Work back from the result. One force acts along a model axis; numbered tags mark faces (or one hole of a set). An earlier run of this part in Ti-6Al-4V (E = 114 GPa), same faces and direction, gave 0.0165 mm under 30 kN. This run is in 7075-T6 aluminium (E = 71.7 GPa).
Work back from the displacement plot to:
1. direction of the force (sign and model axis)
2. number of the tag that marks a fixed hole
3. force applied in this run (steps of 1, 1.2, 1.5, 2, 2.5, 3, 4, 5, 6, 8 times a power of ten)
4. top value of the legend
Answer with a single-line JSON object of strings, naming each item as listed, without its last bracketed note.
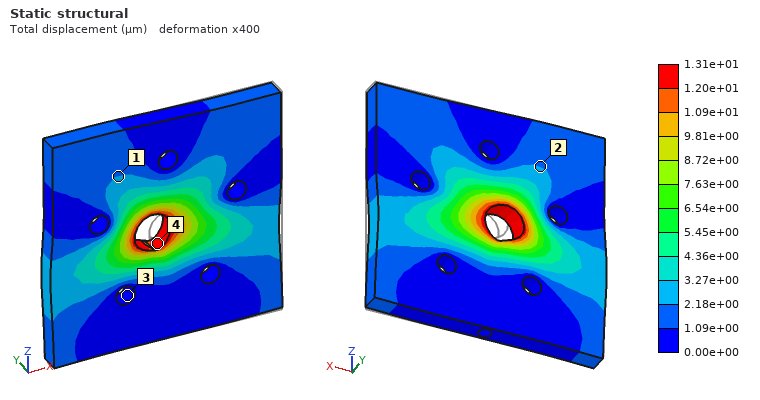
{"direction of the force": "-X", "number of the tag that marks a fixed hole": "3", "force applied in this run": "15 kN", "top value of the legend": "1.31e+01 µm"}
